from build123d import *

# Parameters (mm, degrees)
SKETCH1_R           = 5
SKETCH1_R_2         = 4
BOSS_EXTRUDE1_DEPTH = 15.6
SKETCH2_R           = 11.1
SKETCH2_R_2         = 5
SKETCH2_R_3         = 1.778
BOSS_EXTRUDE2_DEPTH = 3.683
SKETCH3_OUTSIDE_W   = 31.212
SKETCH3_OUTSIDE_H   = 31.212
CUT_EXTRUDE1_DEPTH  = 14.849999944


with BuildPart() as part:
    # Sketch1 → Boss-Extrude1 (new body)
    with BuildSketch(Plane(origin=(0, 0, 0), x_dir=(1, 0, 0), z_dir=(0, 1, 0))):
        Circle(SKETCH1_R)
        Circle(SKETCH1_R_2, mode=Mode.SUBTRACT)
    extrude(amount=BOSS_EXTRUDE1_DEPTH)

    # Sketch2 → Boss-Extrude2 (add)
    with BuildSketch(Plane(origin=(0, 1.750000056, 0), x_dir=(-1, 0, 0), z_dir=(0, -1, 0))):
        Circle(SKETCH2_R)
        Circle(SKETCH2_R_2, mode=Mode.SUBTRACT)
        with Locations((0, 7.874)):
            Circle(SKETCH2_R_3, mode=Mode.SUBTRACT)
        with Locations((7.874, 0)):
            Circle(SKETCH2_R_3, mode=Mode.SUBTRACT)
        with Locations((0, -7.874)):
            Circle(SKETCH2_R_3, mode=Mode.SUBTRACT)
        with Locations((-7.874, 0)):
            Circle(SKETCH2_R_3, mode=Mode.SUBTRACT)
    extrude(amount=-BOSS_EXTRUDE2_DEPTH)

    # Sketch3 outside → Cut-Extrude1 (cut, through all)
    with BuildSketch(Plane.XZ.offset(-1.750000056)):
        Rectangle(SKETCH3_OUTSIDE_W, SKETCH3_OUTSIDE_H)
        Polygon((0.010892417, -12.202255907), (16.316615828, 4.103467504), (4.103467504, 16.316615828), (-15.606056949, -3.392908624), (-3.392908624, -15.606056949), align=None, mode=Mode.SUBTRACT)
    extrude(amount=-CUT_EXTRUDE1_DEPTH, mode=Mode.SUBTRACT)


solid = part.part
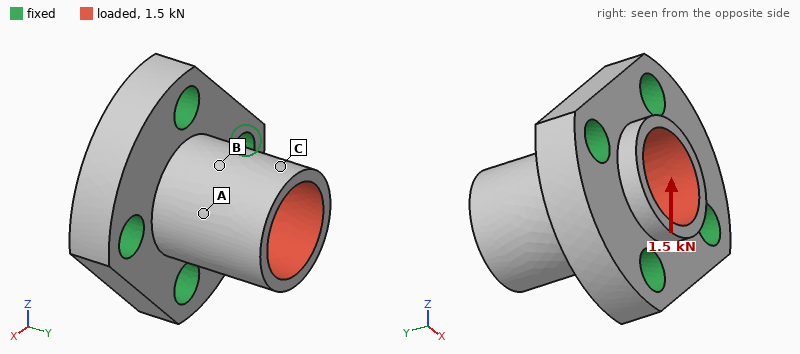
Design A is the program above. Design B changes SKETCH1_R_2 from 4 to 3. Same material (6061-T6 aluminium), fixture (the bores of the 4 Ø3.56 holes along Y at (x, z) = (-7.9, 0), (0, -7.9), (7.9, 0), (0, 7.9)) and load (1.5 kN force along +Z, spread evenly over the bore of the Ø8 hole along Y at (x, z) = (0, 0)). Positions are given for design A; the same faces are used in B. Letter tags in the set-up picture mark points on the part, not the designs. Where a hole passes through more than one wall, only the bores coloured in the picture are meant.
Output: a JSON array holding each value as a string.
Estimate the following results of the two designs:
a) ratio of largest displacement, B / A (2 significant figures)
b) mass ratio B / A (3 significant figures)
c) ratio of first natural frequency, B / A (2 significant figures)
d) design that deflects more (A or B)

["0.64", "1.27", "0.95", "A"]
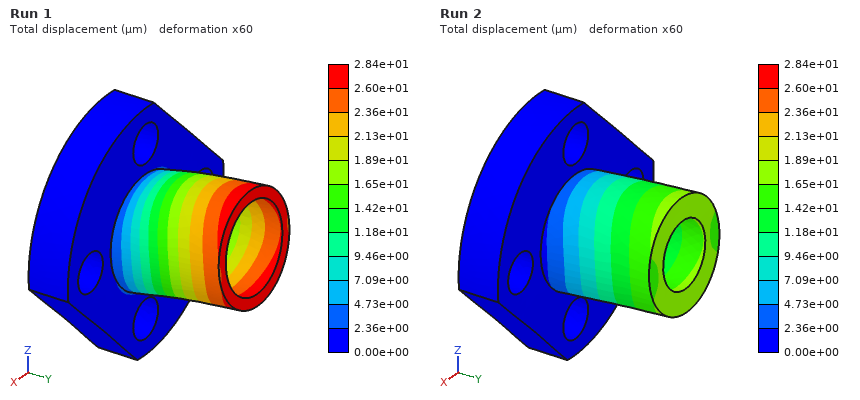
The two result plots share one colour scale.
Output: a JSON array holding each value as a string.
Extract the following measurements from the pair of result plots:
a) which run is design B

["Run 2"]
